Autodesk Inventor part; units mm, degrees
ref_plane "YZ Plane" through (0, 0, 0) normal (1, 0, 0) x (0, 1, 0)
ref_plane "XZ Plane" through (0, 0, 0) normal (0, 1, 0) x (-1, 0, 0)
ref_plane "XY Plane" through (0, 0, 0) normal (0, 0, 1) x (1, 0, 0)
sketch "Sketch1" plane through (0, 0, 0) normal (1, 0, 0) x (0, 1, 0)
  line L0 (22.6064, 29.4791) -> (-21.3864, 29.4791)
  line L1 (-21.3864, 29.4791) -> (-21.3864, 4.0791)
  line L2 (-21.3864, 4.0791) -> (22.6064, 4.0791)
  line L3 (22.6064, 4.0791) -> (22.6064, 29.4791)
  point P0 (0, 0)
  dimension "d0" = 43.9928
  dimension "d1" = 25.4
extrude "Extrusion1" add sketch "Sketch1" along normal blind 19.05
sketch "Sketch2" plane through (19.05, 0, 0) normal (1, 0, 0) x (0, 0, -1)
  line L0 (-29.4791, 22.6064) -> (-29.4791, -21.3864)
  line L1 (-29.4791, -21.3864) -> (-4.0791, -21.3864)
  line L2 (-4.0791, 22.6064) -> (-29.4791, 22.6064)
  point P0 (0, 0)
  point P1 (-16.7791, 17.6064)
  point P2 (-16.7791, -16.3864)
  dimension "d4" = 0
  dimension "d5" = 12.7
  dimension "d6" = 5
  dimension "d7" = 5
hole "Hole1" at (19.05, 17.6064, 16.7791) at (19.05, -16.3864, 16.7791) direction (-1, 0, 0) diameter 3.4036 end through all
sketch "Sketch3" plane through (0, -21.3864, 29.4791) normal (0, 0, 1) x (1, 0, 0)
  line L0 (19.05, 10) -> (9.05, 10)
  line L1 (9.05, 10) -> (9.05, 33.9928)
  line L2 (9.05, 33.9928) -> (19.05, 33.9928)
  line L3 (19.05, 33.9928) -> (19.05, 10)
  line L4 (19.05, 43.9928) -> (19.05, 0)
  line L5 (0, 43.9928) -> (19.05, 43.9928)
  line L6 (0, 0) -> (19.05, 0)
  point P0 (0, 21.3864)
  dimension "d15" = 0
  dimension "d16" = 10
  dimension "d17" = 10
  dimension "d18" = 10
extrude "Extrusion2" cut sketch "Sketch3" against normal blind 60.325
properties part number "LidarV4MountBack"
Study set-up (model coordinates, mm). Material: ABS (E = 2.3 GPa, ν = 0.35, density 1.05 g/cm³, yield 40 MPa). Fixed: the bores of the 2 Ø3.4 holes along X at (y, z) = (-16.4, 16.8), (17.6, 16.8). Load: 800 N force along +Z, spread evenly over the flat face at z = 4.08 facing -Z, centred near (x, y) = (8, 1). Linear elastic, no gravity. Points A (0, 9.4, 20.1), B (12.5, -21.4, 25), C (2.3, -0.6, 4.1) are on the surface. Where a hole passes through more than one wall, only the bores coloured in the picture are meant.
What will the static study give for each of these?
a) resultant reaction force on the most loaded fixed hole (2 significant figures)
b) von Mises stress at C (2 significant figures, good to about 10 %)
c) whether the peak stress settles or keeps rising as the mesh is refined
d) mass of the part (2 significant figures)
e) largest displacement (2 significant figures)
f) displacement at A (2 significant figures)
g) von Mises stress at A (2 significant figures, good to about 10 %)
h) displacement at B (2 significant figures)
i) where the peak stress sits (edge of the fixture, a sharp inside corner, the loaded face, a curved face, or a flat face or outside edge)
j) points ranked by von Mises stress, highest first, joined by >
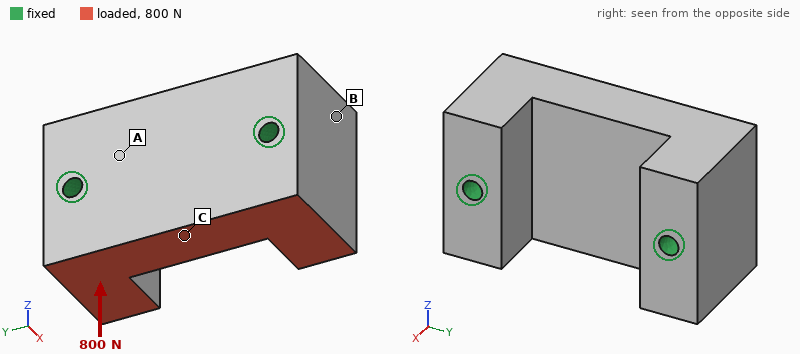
400 N
1.6 MPa
keeps rising
16 g
22 µm
11 µm
1.2 MPa
3.3 µm
edge of the fixture
C > A > B
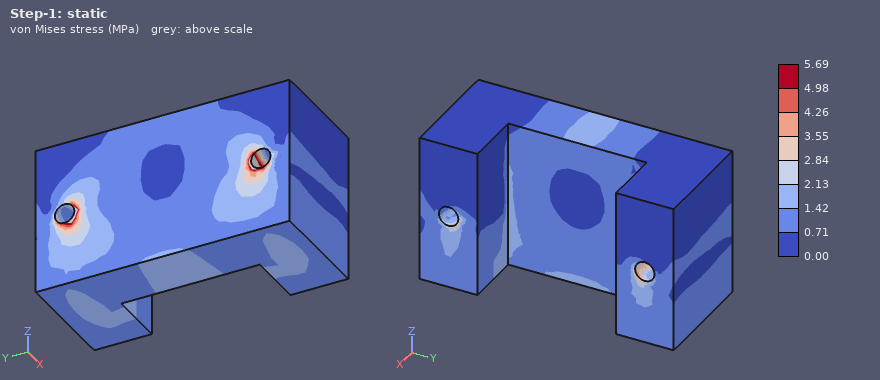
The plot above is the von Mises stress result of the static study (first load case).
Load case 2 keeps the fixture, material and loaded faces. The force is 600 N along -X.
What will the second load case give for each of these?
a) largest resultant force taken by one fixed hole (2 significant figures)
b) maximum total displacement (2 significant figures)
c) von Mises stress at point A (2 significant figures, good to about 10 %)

300 N
81 µm
2.1 MPa
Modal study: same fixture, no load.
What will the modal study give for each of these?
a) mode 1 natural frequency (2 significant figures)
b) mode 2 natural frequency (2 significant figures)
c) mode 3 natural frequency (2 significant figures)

8400 Hz
8400 Hz
9900 Hz
